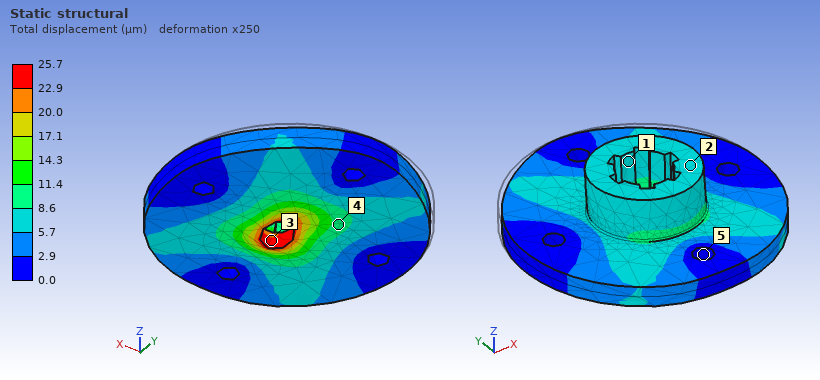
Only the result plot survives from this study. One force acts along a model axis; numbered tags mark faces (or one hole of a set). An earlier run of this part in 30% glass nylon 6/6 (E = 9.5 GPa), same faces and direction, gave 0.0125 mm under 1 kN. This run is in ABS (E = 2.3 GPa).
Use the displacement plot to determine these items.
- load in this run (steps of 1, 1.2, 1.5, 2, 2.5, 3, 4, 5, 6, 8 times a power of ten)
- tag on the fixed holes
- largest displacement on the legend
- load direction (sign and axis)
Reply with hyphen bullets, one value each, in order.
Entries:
- 500 N
- 5
- 25.7 µm
- -Y
